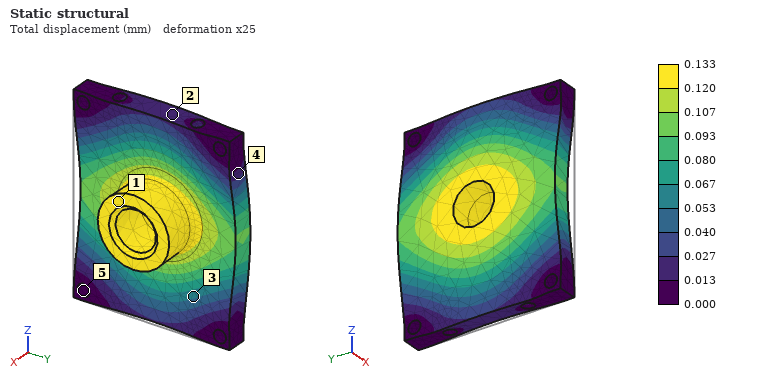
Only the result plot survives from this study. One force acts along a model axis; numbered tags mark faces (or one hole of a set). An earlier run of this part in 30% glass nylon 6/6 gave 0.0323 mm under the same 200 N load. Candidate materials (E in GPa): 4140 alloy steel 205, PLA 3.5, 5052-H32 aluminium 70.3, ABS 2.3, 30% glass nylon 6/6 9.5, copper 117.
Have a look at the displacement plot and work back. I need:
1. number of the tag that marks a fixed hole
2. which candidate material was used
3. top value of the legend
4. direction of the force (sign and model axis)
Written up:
5
ABS
0.133 mm
-X
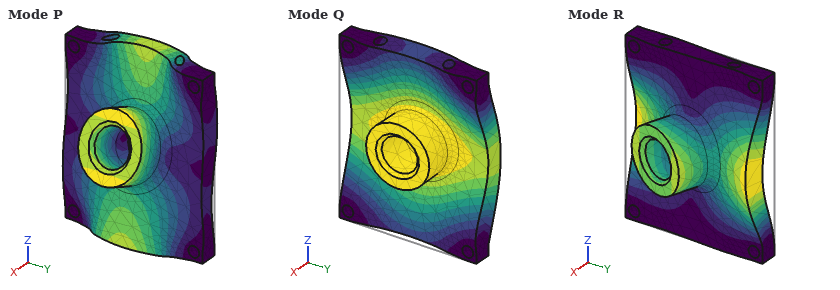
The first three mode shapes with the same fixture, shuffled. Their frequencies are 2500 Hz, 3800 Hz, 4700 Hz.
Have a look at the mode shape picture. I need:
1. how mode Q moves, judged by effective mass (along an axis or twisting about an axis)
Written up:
along X
